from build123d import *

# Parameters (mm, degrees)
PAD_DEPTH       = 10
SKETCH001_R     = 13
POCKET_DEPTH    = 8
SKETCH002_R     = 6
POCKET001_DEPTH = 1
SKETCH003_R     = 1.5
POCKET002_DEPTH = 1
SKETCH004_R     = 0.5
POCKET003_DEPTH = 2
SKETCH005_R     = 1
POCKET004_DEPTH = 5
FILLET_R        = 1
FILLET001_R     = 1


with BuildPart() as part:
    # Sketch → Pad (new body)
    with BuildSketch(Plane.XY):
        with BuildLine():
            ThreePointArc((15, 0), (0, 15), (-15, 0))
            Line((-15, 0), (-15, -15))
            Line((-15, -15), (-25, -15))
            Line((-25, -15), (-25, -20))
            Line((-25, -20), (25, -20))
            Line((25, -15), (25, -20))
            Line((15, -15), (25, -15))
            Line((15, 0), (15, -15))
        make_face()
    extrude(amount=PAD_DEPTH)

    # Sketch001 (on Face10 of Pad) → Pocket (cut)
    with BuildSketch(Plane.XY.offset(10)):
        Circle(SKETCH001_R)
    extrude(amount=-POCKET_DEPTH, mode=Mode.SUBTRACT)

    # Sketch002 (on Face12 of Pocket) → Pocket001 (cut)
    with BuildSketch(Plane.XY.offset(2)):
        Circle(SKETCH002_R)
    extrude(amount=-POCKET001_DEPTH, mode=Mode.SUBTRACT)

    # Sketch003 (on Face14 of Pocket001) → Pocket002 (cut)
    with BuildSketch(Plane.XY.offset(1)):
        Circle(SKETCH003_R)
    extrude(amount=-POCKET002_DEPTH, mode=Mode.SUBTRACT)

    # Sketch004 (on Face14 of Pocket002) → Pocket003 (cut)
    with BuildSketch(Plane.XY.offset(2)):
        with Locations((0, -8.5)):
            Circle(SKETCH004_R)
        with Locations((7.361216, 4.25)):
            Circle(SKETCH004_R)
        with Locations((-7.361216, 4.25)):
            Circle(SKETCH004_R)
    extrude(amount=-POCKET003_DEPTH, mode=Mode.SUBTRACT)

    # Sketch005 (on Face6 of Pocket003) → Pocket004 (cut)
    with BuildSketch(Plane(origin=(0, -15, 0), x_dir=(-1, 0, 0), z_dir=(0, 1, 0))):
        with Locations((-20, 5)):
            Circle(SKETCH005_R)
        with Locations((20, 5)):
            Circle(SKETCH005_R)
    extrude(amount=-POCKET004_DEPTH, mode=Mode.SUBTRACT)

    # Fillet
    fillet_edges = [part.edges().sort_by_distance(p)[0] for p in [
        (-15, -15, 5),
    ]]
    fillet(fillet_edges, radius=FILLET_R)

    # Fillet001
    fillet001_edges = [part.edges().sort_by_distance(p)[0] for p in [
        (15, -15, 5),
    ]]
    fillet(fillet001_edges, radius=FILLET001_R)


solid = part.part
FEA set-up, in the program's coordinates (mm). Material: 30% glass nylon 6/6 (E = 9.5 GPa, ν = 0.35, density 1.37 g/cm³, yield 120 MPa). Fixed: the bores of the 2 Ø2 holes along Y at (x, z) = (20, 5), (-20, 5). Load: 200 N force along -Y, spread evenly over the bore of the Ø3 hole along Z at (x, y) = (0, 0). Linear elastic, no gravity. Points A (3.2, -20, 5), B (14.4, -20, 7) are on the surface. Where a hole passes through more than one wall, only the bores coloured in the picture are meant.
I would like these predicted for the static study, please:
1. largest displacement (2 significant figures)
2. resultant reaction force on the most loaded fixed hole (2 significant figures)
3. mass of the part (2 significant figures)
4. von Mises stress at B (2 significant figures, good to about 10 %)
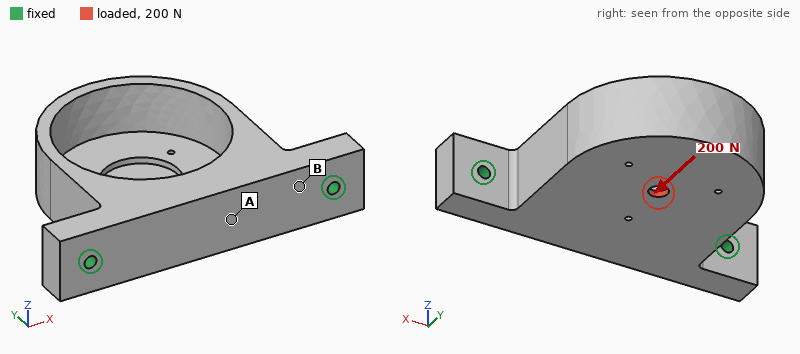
0.13 mm
110 N
8.4 g
5.3 MPa
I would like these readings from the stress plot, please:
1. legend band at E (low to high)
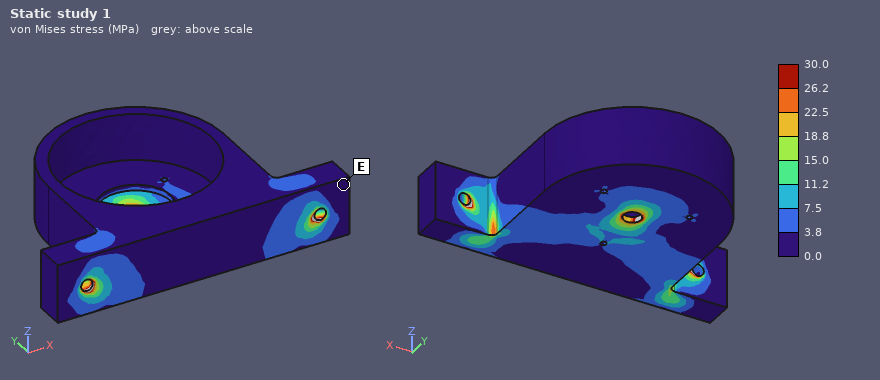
0.0 to 3.8 MPa
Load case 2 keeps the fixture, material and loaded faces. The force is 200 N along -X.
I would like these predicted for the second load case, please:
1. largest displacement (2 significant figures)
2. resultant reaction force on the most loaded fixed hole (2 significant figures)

45 µm
140 N
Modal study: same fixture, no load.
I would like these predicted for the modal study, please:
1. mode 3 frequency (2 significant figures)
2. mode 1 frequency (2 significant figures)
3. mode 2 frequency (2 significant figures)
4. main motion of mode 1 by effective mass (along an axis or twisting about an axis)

7100 Hz
1900 Hz
4600 Hz
along Z
